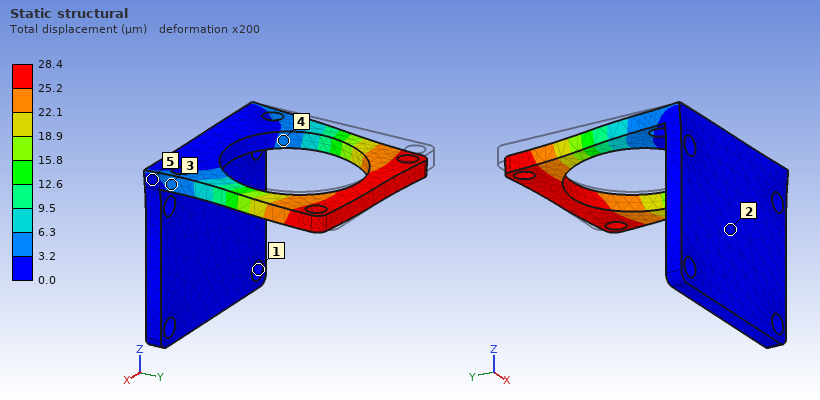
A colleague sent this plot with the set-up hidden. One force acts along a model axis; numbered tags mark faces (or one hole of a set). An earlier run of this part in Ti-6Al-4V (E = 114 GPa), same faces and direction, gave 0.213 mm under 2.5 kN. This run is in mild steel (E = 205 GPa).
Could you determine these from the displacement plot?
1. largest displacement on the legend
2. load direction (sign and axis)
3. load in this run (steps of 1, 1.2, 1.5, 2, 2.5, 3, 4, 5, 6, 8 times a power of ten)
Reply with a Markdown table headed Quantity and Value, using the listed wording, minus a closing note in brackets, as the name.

| Quantity | Value |
|---|---|
| largest displacement on the legend | 28.4 µm |
| load direction | +X |
| load in this run | 600 N |
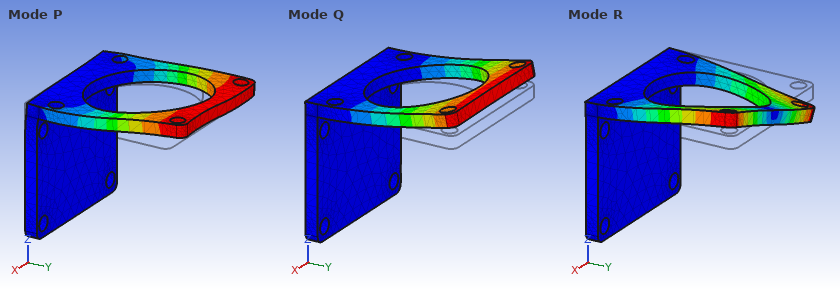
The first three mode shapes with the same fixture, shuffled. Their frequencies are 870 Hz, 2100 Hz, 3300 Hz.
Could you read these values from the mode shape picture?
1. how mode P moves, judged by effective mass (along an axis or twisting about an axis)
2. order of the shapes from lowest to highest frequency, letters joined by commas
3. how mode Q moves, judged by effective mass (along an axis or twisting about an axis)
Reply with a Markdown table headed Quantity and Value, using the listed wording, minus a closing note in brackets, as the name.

| Quantity | Value |
|---|---|
| how mode P moves, judged by effective mass | along X |
| order of the shapes from lowest to highest frequency, letters joined by commas | Q, R, P |
| how mode Q moves, judged by effective mass | along Z |
